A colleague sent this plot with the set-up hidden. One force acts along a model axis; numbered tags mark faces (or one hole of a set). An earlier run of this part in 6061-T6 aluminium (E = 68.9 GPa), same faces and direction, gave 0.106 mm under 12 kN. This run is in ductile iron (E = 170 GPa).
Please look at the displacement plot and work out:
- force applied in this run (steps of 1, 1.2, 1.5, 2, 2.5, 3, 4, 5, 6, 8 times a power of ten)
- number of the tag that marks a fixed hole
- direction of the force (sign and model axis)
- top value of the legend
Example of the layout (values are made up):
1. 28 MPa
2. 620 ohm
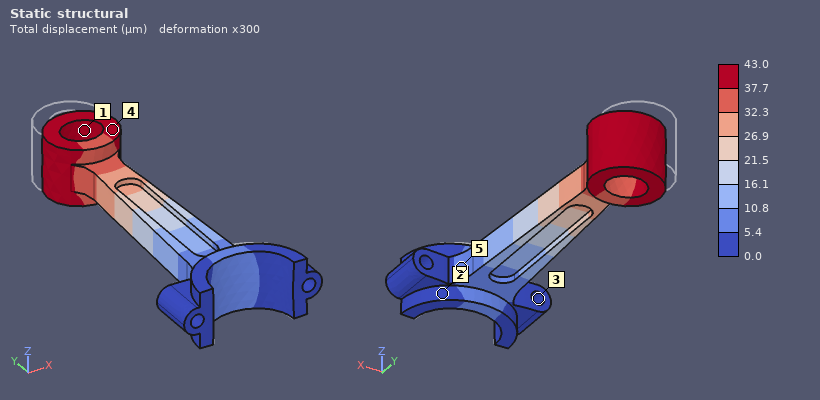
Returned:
1. 12 kN
2. 3
3. -Y
4. 43.0 µm
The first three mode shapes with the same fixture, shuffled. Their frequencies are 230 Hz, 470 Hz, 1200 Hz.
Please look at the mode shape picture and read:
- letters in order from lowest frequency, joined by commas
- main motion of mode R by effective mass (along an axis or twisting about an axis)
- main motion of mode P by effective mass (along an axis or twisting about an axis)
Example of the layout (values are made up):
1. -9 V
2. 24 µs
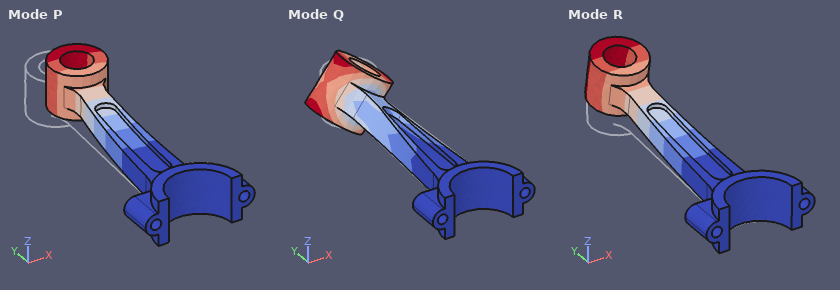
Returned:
1. R, P, Q
2. along Z
3. along X
